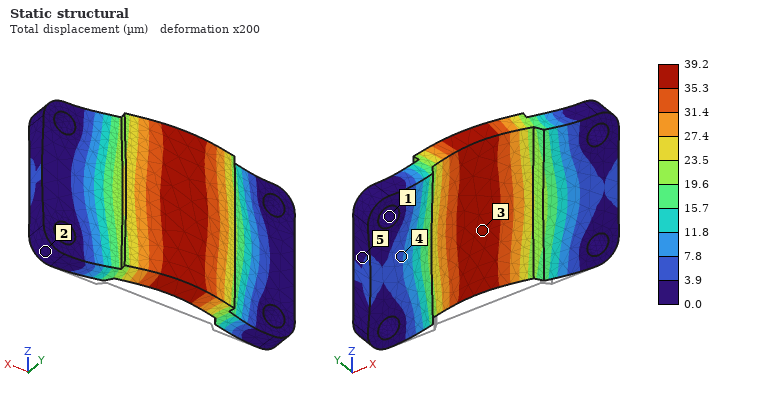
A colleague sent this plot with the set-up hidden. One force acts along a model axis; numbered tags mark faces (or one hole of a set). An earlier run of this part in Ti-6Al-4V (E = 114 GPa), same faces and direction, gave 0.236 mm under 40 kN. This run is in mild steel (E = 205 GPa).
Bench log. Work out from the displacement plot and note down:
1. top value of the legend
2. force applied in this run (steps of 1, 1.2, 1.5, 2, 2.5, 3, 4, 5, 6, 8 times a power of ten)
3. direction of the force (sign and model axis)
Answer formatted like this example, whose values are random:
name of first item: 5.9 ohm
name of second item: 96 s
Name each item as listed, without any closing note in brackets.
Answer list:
top value of the legend: 39.2 µm
force applied in this run: 12 kN
direction of the force: +Y
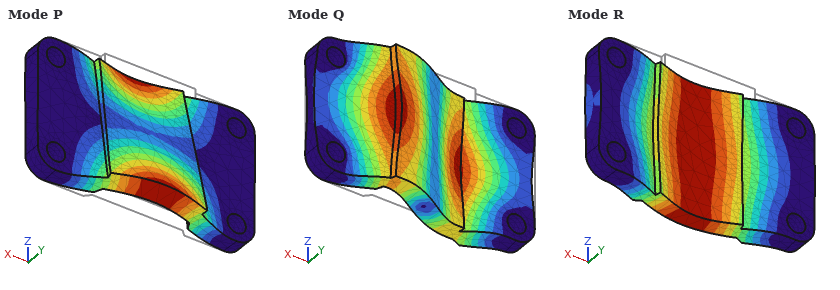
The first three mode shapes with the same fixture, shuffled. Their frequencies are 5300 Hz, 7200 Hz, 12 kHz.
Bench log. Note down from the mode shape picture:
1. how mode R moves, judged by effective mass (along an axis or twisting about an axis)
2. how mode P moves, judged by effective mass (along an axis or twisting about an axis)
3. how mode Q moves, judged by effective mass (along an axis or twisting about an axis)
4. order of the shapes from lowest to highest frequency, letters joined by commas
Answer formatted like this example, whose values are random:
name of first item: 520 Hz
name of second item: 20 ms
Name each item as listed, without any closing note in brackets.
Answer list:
how mode R moves, judged by effective mass: along Y
how mode P moves, judged by effective mass: twisting about X
how mode Q moves, judged by effective mass: twisting about Z
order of the shapes from lowest to highest frequency, letters joined by commas: R, P, Q
